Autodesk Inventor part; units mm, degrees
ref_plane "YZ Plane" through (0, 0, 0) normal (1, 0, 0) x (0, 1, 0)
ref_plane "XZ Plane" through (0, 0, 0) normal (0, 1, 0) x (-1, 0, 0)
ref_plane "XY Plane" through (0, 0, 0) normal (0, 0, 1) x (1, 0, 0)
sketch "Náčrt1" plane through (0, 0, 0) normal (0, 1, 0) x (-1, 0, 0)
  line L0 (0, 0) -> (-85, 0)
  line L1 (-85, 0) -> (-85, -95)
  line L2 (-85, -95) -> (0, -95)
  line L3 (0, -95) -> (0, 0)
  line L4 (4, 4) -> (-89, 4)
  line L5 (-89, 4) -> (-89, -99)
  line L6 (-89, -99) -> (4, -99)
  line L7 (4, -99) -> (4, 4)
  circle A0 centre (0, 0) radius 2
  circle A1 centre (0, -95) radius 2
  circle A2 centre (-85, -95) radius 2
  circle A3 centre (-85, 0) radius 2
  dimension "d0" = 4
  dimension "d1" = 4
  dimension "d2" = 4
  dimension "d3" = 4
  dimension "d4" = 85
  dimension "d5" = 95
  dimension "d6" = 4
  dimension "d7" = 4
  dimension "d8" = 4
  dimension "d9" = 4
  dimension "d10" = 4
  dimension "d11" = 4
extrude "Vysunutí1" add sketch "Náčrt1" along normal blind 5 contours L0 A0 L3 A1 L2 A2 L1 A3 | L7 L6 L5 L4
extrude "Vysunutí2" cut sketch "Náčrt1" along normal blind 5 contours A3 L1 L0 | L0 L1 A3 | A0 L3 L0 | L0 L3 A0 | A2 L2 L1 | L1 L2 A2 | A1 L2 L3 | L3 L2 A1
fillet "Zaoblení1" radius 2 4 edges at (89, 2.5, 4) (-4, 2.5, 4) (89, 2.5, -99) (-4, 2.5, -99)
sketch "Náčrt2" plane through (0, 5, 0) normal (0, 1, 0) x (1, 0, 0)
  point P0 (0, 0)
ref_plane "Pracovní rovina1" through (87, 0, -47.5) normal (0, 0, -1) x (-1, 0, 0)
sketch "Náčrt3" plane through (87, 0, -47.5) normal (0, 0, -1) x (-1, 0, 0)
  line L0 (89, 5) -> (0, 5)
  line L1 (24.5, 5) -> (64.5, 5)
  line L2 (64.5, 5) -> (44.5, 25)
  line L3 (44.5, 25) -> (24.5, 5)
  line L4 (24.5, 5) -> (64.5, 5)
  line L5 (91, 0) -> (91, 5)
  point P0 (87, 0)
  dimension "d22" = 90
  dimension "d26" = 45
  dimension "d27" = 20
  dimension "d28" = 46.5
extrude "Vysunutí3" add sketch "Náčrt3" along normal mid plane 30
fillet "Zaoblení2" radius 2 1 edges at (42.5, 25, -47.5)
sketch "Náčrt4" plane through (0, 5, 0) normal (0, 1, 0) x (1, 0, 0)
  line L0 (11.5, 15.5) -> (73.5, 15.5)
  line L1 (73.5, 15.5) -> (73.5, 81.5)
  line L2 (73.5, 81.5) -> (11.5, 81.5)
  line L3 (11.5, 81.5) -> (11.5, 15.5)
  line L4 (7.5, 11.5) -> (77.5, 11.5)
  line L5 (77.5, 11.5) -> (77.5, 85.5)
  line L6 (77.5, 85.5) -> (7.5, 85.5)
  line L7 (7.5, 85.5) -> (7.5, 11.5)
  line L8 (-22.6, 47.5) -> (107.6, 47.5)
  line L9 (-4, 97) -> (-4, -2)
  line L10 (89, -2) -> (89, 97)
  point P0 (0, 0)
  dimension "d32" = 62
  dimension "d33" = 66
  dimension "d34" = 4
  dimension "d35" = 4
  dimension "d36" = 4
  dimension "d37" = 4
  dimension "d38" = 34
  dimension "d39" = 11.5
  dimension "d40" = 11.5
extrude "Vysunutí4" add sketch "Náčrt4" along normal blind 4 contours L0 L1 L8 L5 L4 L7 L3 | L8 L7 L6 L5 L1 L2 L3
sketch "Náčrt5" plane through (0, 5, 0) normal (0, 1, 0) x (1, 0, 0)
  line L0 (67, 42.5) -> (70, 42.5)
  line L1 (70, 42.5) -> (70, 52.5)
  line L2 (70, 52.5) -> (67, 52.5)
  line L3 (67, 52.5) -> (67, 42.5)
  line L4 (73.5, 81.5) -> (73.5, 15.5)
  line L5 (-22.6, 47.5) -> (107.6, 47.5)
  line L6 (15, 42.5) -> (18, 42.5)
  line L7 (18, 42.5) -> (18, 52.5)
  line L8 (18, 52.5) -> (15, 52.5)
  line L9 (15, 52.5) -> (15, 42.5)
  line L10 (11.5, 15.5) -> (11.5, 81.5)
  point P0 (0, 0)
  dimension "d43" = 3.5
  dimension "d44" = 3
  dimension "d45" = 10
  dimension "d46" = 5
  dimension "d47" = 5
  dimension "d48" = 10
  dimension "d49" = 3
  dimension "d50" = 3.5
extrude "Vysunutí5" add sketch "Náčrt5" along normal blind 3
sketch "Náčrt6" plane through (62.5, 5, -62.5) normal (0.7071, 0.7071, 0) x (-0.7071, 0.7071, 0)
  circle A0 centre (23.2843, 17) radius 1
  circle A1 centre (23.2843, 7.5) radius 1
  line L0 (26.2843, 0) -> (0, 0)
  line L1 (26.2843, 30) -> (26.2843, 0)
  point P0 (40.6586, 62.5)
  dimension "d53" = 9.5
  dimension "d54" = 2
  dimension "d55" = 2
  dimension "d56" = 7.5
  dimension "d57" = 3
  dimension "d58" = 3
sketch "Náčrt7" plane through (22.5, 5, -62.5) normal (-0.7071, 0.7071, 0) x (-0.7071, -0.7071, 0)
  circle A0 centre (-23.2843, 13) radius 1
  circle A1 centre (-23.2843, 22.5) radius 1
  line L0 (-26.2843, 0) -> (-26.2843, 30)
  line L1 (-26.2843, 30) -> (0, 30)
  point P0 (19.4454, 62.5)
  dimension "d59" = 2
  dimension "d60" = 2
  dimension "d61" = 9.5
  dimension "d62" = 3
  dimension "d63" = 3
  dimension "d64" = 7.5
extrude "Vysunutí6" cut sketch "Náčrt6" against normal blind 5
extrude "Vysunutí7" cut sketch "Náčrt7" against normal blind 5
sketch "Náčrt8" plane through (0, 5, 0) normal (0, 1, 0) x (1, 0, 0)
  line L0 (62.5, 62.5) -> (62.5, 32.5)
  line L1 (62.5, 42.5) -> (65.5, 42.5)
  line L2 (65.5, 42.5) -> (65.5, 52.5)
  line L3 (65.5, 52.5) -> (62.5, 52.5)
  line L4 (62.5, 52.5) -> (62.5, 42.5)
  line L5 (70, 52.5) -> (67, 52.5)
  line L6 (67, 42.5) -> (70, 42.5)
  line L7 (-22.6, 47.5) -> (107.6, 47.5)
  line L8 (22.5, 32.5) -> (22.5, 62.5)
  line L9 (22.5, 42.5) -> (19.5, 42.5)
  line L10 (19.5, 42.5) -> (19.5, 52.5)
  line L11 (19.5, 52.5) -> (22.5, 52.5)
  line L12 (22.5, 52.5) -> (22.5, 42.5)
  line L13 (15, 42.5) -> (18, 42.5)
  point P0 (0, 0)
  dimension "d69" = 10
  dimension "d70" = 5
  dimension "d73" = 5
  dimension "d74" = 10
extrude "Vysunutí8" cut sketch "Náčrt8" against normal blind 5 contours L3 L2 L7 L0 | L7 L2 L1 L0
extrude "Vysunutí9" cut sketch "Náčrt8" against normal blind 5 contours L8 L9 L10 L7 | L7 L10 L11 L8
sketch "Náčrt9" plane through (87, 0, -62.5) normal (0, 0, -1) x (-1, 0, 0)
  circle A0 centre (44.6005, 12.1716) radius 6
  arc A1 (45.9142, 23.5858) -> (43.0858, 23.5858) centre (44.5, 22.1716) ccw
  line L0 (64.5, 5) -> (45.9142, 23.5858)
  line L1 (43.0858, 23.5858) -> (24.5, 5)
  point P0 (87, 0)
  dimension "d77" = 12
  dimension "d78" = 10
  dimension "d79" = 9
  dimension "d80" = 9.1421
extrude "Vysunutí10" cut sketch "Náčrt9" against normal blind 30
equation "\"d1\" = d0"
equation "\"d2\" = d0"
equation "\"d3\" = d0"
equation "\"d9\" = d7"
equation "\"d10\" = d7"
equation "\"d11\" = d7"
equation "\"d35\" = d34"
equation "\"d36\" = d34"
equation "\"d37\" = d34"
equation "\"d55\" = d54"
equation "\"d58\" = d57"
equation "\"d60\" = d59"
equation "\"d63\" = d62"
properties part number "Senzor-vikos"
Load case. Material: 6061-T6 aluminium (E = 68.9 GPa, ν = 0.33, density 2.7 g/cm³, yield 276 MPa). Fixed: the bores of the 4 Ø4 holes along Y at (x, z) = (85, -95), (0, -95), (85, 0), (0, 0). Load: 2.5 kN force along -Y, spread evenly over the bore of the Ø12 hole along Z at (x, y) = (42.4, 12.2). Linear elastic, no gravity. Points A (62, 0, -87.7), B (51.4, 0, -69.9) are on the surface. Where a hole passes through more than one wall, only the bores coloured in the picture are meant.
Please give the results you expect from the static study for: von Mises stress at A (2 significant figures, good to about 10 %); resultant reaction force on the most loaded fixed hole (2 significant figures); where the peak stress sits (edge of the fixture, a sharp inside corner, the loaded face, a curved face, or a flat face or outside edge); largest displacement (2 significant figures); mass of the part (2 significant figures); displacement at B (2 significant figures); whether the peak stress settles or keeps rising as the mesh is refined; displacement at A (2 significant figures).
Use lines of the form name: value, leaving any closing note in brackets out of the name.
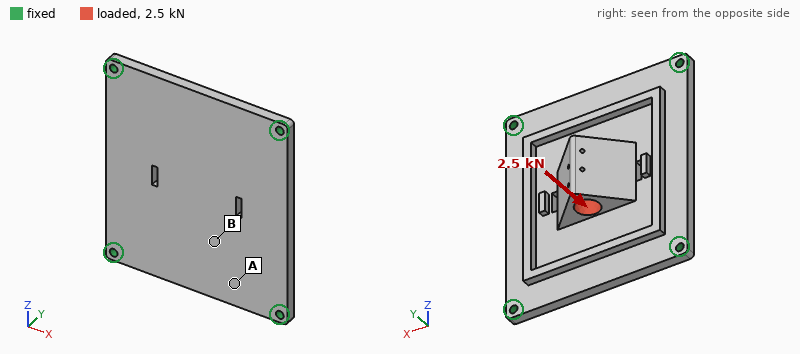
von Mises stress at A: 17 MPa
resultant reaction force on the most loaded fixed hole: 800 N
where the peak stress sits: edge of the fixture
largest displacement: 0.20 mm
mass of the part: 160 g
displacement at B: 0.18 mm
whether the peak stress settles or keeps rising as the mesh is refined: keeps rising
displacement at A: 0.083 mm
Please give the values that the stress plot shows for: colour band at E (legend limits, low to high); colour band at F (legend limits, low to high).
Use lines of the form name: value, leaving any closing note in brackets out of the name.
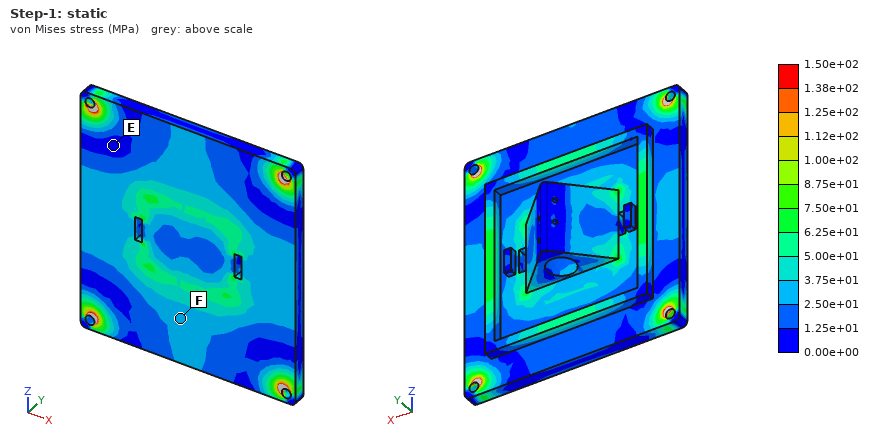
colour band at E: 0.00e+00 to 1.25e+01 MPa
colour band at F: 2.50e+01 to 3.75e+01 MPa
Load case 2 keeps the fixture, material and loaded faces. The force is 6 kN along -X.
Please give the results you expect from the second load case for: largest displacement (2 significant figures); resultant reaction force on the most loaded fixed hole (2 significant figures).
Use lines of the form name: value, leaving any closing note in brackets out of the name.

largest displacement: 97 µm
resultant reaction force on the most loaded fixed hole: 1.9 kN
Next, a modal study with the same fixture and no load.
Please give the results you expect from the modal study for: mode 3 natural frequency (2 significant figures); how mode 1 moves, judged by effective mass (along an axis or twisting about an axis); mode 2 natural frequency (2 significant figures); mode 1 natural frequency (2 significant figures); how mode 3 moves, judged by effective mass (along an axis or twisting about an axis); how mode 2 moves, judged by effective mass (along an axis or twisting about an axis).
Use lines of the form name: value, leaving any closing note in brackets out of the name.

mode 3 natural frequency: 3700 Hz
how mode 1 moves, judged by effective mass: along Y
mode 2 natural frequency: 3300 Hz
mode 1 natural frequency: 1900 Hz
how mode 3 moves, judged by effective mass: twisting about X
how mode 2 moves, judged by effective mass: twisting about Z
